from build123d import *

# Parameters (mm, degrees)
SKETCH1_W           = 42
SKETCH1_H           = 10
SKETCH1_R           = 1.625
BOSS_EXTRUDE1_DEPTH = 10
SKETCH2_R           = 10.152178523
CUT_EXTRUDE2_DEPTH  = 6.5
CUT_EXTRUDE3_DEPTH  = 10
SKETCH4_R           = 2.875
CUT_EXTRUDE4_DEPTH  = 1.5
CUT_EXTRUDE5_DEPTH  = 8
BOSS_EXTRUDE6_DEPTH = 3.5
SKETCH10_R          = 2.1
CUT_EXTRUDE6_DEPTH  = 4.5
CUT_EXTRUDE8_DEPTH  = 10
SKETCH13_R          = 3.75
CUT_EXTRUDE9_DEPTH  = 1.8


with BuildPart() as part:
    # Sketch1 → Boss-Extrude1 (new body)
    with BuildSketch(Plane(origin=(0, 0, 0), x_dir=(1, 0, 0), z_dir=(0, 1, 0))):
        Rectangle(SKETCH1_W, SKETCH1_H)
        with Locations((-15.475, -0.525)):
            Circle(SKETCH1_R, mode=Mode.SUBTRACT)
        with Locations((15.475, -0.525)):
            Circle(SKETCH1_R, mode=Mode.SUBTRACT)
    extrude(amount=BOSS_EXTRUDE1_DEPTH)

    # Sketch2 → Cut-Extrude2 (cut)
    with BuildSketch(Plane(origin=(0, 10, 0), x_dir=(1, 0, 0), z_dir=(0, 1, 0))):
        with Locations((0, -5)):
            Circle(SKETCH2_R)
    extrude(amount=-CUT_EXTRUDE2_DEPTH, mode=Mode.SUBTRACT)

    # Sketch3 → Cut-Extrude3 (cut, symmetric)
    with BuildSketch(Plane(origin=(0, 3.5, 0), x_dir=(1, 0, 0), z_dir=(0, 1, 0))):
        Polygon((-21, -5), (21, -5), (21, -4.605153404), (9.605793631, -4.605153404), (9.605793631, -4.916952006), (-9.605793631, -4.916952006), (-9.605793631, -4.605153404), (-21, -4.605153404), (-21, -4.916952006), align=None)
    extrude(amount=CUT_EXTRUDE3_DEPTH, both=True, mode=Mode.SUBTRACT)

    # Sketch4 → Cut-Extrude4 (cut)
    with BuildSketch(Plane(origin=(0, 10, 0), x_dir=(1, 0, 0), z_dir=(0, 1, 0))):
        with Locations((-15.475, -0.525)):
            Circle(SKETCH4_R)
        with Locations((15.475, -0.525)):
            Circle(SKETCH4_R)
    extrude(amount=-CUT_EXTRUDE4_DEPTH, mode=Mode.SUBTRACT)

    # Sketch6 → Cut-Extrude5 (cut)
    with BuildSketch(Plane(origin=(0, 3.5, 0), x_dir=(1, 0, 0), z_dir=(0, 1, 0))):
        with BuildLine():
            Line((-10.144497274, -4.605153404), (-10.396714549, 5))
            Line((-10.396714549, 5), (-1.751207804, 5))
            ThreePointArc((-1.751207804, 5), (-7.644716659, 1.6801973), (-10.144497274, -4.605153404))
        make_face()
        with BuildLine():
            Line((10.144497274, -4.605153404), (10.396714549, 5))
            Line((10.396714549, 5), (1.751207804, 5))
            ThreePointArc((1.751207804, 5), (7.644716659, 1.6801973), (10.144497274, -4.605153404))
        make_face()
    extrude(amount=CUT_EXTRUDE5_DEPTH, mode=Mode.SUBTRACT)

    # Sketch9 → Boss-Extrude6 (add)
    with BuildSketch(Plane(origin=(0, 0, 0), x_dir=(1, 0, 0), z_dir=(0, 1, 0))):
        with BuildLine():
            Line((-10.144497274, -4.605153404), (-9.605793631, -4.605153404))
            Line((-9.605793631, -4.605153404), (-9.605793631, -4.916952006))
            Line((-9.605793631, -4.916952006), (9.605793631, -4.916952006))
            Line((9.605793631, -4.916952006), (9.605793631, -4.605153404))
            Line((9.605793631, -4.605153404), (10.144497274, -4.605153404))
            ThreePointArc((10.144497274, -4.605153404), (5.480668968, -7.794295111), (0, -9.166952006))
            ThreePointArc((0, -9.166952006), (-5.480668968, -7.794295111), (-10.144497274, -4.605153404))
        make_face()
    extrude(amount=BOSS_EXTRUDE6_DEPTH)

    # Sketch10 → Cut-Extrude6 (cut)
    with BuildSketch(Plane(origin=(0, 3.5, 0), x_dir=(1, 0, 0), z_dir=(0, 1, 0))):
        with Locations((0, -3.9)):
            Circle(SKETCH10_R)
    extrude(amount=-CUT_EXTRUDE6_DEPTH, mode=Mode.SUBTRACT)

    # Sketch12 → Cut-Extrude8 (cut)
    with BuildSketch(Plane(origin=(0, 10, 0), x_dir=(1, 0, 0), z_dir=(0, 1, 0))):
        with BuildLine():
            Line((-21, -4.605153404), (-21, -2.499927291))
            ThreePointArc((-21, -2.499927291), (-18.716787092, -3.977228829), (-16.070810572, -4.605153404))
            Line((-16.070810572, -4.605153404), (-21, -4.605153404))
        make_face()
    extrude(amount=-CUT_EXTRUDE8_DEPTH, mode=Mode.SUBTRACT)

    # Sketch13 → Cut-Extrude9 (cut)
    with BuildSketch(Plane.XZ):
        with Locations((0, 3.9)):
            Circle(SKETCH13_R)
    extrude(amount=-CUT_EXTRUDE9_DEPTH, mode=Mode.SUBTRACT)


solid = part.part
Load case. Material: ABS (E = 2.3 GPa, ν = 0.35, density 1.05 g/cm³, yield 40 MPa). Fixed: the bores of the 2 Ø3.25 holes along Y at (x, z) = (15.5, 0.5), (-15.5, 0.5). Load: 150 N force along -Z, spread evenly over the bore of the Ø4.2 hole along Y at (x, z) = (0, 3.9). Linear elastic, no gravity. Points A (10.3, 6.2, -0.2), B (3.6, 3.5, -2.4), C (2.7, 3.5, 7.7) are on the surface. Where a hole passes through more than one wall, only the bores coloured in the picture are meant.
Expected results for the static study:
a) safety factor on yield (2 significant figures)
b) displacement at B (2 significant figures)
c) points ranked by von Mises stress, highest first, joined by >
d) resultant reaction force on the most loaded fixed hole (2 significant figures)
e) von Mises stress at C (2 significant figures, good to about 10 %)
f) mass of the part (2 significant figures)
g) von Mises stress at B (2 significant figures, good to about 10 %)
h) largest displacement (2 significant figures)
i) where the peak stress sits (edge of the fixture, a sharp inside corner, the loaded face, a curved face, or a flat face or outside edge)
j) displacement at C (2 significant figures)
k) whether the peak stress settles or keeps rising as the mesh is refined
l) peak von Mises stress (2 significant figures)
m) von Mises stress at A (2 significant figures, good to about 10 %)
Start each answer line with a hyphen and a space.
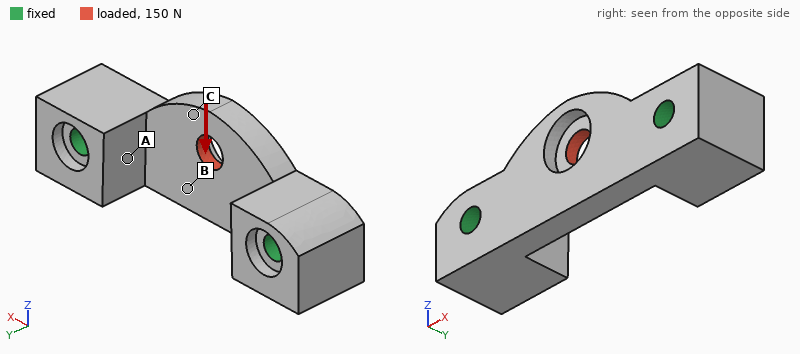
- 3.1
- 54 µm
- C > B > A
- 76 N
- 7.2 MPa
- 2.7 g
- 4.8 MPa
- 88 µm
- a curved face
- 75 µm
- settles
- 13 MPa
- 1.9 MPa
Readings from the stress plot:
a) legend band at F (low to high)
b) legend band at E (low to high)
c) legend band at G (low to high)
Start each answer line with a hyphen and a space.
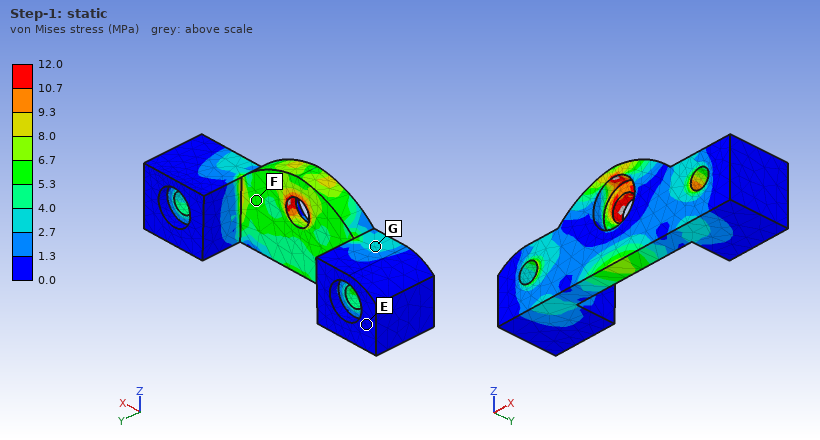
- 5.3 to 6.7 MPa
- 0.0 to 1.3 MPa
- 2.7 to 4.0 MPa
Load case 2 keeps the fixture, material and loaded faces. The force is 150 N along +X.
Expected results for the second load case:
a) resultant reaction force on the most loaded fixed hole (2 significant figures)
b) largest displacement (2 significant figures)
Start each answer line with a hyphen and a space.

- 77 N
- 31 µm
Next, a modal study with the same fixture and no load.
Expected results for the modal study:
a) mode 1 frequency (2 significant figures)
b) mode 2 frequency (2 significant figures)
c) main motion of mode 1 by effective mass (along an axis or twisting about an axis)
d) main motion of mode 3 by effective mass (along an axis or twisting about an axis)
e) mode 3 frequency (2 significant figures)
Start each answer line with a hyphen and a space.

- 6900 Hz
- 9400 Hz
- along Y
- along Z
- 11 kHz
